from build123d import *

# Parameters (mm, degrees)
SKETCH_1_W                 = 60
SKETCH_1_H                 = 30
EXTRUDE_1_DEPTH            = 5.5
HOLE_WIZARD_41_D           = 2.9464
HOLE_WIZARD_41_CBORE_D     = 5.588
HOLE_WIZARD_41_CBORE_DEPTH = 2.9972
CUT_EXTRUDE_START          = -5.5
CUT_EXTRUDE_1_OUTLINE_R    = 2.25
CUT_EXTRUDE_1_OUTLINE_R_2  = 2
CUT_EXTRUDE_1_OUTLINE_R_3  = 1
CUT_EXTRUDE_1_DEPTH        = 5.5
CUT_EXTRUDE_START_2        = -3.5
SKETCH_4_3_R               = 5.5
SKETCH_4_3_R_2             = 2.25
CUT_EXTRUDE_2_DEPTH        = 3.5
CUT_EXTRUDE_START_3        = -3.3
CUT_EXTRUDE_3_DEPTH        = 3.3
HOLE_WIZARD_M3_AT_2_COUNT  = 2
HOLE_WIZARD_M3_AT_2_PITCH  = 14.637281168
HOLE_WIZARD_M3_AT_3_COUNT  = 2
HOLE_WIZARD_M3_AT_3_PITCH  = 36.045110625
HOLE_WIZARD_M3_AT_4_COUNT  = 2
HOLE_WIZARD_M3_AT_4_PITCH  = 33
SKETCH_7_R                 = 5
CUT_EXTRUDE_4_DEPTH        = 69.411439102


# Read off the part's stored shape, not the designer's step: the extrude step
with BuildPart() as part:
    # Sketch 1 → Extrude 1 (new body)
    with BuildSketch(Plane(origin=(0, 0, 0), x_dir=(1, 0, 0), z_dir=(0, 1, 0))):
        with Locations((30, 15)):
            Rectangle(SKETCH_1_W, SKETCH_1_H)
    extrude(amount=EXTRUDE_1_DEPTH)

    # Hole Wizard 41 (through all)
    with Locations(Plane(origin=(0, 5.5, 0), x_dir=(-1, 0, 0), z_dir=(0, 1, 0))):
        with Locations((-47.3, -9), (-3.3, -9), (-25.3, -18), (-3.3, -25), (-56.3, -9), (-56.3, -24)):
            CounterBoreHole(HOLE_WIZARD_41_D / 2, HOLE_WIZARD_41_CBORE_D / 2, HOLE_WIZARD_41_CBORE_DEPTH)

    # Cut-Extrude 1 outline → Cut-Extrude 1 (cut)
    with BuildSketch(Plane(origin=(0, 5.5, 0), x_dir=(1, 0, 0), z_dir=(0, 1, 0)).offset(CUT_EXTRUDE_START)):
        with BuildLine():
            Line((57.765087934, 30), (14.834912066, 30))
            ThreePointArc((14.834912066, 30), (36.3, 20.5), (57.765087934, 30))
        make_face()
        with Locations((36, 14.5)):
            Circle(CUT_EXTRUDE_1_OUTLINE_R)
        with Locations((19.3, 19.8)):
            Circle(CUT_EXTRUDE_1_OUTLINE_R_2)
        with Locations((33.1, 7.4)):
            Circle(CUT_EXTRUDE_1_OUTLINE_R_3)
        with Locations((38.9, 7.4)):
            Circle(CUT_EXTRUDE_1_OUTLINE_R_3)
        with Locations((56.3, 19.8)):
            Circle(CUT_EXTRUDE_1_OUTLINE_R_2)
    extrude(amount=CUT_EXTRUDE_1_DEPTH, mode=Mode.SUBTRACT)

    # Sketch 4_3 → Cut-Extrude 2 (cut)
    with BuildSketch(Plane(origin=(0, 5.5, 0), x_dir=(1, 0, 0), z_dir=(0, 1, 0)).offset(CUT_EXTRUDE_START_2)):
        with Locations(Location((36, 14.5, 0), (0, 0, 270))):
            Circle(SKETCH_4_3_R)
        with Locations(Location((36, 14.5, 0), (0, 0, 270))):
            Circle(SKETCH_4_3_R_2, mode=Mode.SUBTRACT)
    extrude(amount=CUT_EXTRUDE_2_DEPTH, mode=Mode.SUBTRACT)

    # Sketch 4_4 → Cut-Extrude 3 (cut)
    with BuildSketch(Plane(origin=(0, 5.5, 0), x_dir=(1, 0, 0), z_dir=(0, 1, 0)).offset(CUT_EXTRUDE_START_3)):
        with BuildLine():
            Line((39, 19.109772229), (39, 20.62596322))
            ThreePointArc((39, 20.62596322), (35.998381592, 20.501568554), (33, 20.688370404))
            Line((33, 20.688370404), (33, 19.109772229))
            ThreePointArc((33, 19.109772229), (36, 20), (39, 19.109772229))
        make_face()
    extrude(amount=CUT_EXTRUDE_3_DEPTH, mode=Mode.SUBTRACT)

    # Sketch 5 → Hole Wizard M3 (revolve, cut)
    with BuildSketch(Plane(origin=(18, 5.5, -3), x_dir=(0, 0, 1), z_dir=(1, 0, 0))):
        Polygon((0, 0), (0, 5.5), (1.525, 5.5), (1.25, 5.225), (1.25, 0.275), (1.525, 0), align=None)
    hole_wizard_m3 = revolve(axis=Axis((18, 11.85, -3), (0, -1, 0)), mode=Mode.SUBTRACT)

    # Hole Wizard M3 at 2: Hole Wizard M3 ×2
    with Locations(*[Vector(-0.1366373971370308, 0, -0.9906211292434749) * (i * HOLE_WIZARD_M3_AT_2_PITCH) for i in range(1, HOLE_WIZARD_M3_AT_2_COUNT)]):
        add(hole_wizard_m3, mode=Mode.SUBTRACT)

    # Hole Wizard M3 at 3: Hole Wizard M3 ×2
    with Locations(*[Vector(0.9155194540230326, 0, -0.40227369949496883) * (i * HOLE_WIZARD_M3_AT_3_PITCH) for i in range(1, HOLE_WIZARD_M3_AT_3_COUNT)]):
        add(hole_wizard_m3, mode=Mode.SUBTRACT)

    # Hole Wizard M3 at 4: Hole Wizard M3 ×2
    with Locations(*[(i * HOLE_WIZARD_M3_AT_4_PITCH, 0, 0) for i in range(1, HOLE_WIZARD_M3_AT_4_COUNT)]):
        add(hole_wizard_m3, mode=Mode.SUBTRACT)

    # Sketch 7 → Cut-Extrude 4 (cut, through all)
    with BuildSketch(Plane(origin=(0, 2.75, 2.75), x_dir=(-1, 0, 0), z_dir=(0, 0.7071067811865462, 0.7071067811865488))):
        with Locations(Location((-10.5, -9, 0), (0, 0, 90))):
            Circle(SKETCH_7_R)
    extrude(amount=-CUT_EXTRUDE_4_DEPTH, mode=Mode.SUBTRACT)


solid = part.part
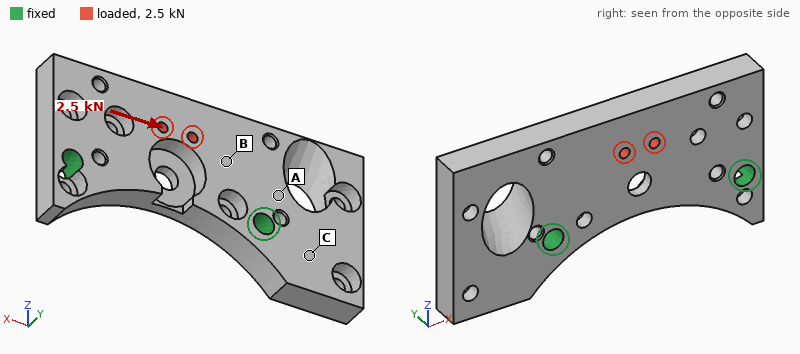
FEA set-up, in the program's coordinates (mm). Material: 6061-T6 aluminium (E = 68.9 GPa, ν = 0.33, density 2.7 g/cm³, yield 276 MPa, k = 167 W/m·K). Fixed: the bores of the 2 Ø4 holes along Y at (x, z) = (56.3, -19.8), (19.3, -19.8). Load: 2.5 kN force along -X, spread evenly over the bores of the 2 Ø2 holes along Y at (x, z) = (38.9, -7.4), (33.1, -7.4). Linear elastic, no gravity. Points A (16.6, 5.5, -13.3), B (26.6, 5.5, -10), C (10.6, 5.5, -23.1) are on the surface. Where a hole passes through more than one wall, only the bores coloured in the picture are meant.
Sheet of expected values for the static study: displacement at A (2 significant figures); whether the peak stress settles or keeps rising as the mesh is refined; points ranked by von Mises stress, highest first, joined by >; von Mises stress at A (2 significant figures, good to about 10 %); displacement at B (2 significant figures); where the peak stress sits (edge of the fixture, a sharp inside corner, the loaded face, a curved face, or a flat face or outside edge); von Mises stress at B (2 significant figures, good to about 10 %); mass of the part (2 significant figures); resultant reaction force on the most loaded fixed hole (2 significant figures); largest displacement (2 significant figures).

5.9 µm
keeps rising
B > A > C
17 MPa
10 µm
edge of the fixture
33 MPa
18 g
1.4 kN
18 µm
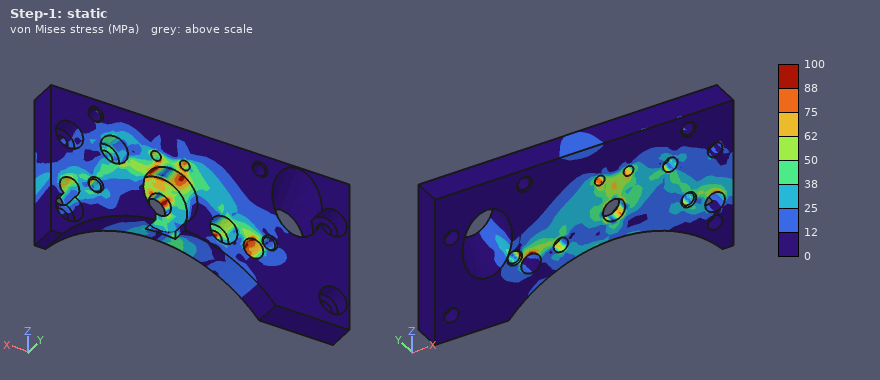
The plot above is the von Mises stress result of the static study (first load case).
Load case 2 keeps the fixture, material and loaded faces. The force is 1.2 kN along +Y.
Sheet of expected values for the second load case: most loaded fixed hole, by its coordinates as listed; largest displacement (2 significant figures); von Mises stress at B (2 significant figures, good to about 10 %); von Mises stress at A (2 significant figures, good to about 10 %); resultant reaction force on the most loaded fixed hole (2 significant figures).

(19.3, -19.8)
0.12 mm
18 MPa
72 MPa
710 N
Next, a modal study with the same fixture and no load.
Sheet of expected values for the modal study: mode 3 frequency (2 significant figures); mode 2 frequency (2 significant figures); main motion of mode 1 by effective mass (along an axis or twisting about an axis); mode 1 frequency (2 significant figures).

12 kHz
8000 Hz
along Y
7100 Hz
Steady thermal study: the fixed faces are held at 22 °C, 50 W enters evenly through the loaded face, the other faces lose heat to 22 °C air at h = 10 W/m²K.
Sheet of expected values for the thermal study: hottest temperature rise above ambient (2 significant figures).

49 K
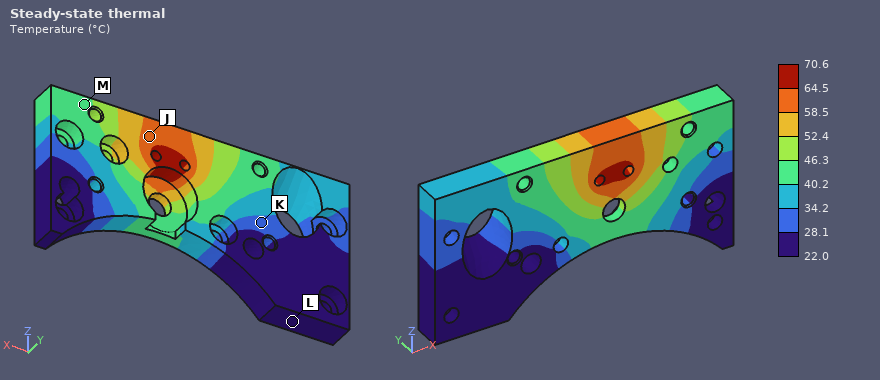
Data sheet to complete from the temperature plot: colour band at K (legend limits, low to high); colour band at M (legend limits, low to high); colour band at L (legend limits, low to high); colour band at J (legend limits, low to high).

28.1 to 34.2 °C
40.2 to 46.3 °C
22.0 to 28.1 °C
58.5 to 64.5 °C
